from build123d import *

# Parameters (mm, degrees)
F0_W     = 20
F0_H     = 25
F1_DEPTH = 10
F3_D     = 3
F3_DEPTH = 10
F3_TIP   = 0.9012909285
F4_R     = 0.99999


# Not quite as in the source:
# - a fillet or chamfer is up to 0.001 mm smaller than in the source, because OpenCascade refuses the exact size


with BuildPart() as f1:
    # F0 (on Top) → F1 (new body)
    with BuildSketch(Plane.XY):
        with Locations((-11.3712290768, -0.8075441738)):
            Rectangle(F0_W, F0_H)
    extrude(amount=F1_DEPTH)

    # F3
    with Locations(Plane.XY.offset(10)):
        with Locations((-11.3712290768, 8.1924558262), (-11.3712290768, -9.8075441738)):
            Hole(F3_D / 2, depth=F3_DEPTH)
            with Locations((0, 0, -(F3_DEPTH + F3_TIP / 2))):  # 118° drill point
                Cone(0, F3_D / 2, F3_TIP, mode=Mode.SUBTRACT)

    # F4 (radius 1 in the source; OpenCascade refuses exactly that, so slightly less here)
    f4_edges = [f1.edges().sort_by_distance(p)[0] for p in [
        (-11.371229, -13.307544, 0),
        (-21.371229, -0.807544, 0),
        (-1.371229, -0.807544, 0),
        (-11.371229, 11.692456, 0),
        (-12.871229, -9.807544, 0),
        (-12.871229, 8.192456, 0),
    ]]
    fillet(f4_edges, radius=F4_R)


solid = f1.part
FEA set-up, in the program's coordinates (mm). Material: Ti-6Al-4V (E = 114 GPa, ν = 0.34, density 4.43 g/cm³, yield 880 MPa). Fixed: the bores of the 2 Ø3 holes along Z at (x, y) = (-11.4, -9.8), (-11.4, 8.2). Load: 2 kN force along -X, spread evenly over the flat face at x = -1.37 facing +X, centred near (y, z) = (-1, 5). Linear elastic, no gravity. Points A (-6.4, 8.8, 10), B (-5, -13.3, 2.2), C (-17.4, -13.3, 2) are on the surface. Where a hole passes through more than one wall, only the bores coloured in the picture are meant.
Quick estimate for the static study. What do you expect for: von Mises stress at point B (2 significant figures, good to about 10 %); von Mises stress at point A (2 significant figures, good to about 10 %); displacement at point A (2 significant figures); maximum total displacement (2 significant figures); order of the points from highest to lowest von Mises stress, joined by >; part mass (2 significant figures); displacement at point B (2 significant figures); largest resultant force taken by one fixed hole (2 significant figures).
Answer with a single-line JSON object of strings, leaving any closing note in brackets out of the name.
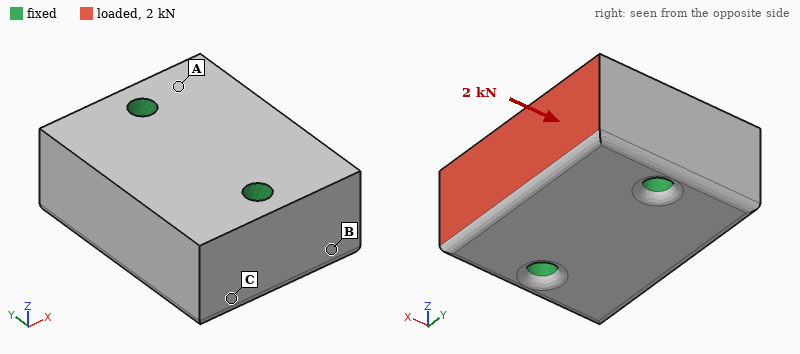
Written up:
{"von Mises stress at point B": "7.2 MPa", "von Mises stress at point A": "12 MPa", "displacement at point A": "0.52 µm", "maximum total displacement": "1.3 µm", "order of the points from highest to lowest von Mises stress, joined by >": "A > B > C", "part mass": "21 g", "displacement at point B": "0.46 µm", "largest resultant force taken by one fixed hole": "1.0 kN"}
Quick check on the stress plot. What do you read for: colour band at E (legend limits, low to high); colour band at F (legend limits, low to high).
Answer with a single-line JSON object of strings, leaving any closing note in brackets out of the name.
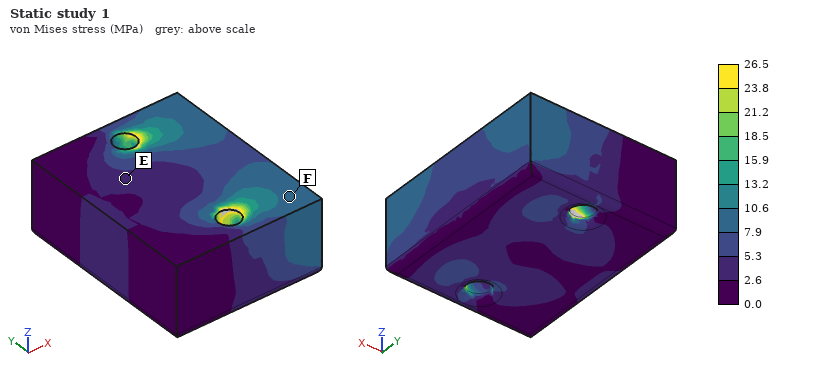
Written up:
{"colour band at E": "2.6 to 5.3 MPa", "colour band at F": "7.9 to 10.6 MPa"}
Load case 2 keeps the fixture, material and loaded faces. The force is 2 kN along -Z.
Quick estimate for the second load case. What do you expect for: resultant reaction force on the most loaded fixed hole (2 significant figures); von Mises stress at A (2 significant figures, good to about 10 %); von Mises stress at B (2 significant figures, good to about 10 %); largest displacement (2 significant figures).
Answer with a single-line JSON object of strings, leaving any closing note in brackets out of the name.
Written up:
{"resultant reaction force on the most loaded fixed hole": "1.0 kN", "von Mises stress at A": "35 MPa", "von Mises stress at B": "19 MPa", "largest displacement": "8.4 µm"}
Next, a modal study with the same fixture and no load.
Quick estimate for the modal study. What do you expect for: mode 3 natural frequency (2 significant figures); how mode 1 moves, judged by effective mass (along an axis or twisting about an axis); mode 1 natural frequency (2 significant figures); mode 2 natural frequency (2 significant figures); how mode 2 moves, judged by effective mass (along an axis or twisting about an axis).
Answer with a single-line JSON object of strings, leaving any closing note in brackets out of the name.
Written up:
{"mode 3 natural frequency": "63 kHz", "how mode 1 moves, judged by effective mass": "twisting about Y", "mode 1 natural frequency": "39 kHz", "mode 2 natural frequency": "46 kHz", "how mode 2 moves, judged by effective mass": "along Z"}
